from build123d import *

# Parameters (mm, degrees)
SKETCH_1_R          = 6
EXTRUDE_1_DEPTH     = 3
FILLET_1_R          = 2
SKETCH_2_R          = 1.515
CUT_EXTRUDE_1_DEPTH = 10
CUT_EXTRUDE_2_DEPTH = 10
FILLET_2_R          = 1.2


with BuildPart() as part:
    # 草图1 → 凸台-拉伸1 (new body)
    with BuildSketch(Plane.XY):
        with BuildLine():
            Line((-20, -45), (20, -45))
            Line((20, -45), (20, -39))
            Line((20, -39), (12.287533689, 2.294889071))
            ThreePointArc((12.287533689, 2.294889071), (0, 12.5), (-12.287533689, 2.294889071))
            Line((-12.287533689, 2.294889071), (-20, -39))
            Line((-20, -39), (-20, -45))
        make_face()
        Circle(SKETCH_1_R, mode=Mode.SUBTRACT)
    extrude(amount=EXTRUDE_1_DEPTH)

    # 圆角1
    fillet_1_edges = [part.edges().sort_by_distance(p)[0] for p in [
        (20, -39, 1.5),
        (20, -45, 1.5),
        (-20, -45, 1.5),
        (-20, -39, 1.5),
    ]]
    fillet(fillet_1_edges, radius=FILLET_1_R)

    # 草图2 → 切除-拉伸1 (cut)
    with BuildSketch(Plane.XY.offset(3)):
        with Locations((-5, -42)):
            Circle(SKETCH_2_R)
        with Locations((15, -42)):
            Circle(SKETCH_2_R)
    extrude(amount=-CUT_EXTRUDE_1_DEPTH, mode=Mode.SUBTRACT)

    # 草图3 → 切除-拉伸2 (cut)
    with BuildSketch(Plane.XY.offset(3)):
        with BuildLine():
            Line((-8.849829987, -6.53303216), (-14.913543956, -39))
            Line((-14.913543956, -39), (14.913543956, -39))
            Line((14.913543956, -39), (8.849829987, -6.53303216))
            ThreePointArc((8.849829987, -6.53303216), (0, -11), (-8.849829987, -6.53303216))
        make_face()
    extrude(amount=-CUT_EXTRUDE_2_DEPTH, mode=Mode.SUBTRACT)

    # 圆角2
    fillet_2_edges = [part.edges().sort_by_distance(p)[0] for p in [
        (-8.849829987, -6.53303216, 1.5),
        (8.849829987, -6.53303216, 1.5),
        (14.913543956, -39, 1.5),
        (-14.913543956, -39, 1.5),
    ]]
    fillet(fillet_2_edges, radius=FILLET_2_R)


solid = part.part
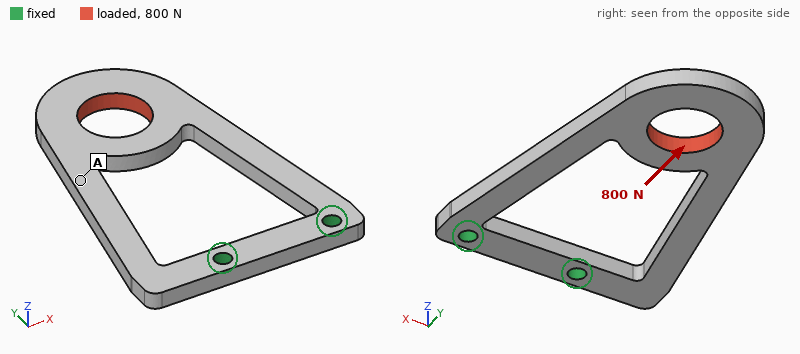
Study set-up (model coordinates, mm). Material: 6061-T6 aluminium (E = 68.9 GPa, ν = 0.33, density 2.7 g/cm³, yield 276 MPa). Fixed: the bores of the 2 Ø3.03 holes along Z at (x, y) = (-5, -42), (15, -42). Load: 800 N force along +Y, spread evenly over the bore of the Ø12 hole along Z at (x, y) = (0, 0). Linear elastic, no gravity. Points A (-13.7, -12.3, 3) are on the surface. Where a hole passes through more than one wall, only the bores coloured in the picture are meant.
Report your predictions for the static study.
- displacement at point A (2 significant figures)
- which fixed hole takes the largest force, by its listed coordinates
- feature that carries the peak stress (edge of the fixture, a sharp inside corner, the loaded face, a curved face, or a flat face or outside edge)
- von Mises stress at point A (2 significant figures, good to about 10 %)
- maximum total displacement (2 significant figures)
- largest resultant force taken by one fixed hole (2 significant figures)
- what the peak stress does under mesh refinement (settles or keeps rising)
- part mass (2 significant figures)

0.11 mm
(-5, -42)
edge of the fixture
27 MPa
0.13 mm
440 N
keeps rising
7.4 g
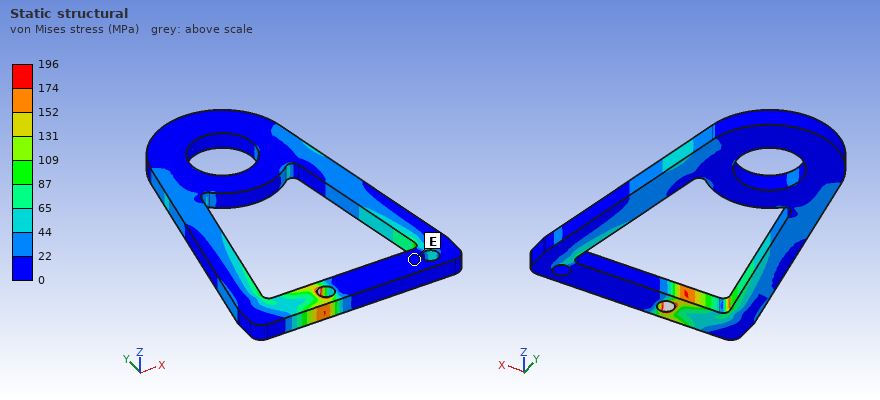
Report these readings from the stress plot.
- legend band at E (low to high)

0 to 22 MPa
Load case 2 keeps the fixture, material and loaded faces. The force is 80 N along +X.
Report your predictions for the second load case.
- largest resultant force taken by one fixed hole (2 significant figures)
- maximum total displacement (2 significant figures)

94 N
82 µm
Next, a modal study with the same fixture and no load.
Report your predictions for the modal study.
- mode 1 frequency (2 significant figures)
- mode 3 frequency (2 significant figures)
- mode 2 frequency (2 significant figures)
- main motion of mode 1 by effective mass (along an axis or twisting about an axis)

610 Hz
2500 Hz
2500 Hz
along Z
